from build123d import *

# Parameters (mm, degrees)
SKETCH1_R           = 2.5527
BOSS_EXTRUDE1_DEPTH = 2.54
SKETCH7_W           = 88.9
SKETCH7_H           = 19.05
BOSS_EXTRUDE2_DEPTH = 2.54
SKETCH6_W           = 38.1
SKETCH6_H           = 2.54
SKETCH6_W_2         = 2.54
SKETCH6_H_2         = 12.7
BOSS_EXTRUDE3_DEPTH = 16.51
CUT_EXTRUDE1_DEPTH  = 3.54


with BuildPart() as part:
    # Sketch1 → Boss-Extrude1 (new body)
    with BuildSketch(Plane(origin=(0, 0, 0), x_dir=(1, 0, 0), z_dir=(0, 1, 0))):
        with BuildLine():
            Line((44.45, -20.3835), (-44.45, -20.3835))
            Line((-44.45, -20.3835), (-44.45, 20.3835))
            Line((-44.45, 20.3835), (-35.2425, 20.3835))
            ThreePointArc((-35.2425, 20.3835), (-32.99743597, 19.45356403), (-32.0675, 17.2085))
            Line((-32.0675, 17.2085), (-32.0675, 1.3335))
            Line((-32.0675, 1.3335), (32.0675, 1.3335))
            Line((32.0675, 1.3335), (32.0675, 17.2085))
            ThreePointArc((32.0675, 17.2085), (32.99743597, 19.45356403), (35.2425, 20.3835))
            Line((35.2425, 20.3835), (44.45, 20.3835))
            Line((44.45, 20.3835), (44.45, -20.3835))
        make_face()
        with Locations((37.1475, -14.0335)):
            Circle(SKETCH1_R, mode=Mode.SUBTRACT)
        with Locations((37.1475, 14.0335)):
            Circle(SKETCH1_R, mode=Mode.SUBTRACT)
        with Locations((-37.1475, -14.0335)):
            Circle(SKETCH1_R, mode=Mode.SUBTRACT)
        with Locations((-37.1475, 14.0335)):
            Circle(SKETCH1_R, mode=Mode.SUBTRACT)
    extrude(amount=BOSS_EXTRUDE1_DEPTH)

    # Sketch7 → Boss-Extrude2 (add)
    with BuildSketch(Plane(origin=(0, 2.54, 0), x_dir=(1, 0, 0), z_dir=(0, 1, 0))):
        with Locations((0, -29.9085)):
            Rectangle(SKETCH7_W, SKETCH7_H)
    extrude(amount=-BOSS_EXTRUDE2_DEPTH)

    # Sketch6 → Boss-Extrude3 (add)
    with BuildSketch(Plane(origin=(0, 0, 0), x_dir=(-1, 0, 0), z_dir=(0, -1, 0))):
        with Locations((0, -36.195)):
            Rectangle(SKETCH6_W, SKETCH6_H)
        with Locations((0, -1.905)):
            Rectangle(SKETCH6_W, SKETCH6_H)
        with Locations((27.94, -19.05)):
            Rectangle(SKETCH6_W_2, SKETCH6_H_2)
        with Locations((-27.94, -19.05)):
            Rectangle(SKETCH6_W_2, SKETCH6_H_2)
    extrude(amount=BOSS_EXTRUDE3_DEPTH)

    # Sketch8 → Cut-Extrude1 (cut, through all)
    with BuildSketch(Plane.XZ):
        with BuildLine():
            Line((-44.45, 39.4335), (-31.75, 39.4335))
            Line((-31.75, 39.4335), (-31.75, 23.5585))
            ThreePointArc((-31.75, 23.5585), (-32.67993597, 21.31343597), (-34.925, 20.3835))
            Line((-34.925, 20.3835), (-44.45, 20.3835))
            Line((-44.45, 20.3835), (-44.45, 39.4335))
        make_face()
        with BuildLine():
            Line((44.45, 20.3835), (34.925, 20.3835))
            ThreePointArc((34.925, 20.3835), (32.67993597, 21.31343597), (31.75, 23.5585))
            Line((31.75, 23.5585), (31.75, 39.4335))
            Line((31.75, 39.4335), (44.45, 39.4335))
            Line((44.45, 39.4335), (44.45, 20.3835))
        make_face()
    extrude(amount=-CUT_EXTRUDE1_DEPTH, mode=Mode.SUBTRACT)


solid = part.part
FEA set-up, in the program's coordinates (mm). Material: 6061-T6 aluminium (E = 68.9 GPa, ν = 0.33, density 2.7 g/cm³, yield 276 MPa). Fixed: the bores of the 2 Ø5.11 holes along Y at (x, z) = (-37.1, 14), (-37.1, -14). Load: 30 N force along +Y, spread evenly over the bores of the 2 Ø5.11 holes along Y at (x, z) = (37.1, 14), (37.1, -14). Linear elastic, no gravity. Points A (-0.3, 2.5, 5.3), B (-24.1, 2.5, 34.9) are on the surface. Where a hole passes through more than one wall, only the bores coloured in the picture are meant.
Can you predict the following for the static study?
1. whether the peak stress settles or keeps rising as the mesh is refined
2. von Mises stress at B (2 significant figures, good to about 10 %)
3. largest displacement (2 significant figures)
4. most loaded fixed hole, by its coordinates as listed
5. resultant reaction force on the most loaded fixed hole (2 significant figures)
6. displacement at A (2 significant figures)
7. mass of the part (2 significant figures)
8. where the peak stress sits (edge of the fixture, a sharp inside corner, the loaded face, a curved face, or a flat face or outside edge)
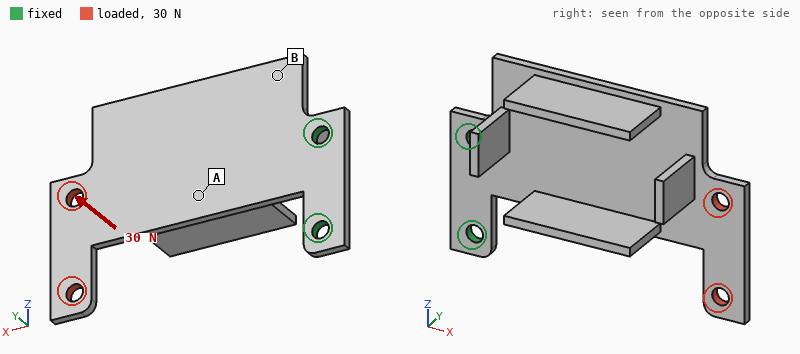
keeps rising
19 MPa
1.3 mm
(-37.1, 14)
38 N
0.40 mm
36 g
edge of the fixture
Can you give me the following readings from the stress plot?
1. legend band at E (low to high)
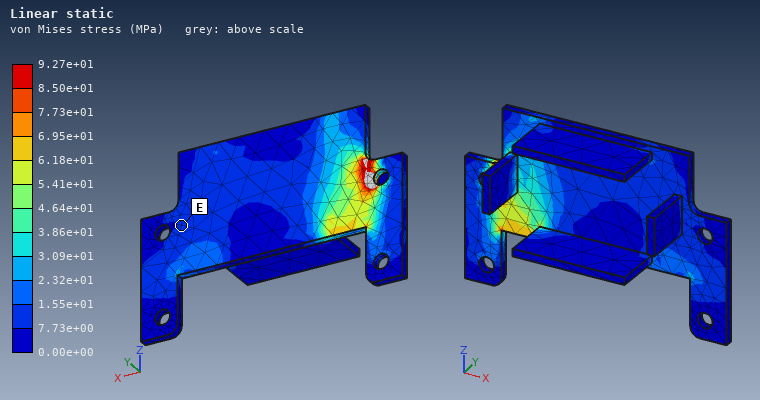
7.73e+00 to 1.55e+01 MPa
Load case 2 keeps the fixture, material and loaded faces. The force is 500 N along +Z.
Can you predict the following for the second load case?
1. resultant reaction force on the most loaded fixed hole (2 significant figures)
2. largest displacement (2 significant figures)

1.2 kN
0.45 mm
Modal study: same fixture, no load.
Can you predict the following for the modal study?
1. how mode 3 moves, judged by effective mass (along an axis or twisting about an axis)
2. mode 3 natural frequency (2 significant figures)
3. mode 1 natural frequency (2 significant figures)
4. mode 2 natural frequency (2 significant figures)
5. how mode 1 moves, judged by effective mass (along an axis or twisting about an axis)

along Z
1600 Hz
270 Hz
740 Hz
along Y
